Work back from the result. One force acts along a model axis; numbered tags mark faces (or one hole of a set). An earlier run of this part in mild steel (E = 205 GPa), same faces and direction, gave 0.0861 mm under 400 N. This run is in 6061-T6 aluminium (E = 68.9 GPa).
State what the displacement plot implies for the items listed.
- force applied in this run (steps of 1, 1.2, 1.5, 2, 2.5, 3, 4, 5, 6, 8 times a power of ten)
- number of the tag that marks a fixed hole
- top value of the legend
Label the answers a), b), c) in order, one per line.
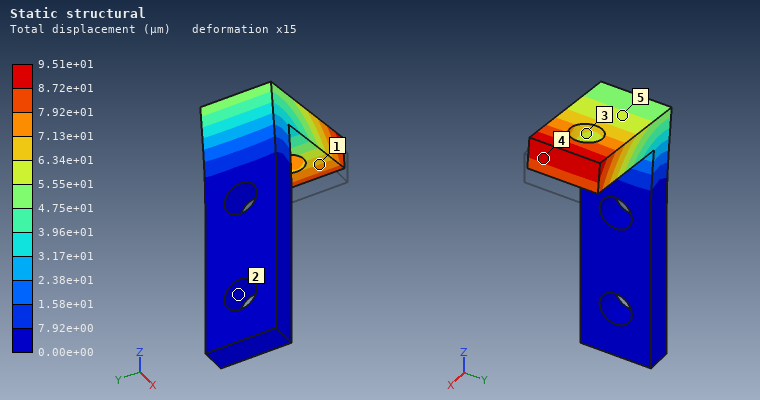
a) 150 N
b) 2
c) 9.51e+01 µm
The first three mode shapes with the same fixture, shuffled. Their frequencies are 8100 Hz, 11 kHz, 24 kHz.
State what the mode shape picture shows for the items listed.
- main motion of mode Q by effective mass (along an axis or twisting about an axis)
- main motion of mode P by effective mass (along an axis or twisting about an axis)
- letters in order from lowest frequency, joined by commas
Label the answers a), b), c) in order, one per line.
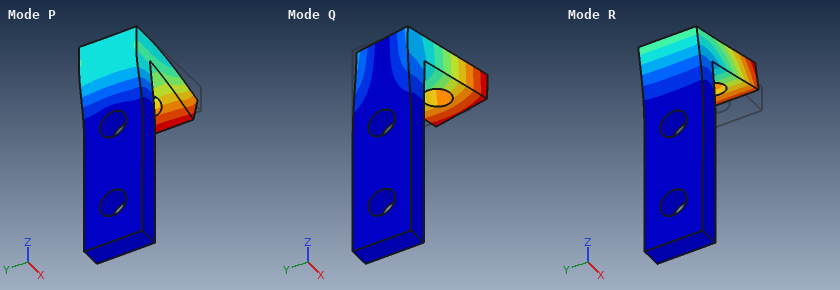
a) along Y
b) along X
c) R, Q, P
